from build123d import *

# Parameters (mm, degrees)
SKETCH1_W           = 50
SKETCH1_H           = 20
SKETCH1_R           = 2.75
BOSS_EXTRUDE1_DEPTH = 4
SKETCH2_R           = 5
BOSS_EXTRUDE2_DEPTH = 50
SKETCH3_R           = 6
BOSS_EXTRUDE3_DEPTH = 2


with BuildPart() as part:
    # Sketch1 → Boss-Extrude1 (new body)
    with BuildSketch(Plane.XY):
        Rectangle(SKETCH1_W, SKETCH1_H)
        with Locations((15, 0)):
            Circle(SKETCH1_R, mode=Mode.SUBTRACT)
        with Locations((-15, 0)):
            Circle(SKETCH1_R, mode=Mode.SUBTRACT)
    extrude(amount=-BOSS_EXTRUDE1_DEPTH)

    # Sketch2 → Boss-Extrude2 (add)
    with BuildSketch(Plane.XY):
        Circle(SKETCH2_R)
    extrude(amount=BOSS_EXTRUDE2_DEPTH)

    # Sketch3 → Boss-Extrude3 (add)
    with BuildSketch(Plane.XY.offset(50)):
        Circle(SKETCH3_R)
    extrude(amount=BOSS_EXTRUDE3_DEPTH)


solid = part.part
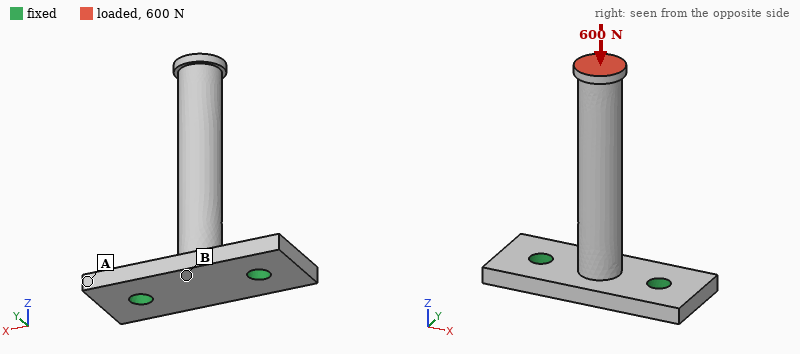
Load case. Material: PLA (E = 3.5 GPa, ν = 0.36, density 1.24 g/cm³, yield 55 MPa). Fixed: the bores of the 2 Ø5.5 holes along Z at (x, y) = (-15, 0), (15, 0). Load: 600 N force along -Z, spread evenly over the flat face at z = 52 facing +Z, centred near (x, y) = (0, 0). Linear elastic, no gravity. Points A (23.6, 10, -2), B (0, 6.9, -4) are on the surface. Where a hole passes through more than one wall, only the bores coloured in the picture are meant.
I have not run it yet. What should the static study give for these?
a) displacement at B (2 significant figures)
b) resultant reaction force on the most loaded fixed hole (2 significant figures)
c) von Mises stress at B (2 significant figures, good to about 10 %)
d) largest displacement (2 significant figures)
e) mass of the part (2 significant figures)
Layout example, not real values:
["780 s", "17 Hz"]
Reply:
["0.16 mm", "310 N", "17 MPa", "0.27 mm", "9.9 g"]
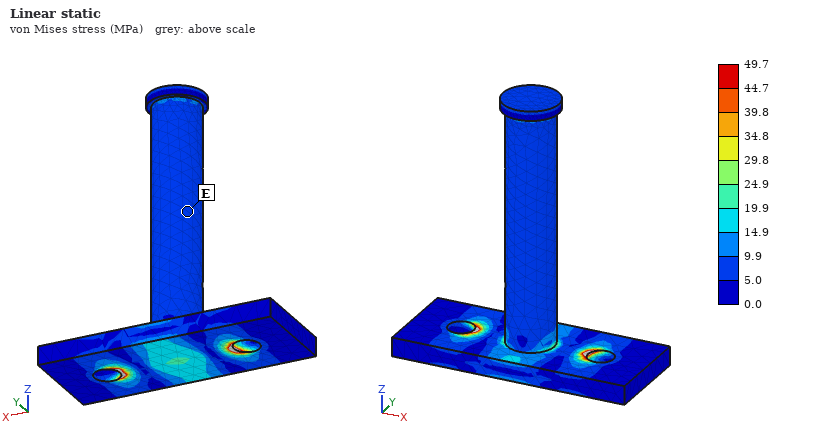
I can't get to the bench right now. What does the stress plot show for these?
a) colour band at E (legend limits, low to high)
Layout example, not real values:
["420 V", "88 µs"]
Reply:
["5.0 to 9.9 MPa"]
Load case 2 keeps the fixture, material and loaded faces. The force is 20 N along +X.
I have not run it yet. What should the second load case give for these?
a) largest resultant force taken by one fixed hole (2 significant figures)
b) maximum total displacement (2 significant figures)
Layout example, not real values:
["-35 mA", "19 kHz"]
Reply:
["55 N", "0.75 mm"]
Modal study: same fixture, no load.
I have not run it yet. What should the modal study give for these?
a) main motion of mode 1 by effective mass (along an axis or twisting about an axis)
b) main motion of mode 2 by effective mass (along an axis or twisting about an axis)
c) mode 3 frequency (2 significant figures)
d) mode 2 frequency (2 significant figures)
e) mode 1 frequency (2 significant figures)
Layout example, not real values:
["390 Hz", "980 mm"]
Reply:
["along Y", "along X", "3600 Hz", "680 Hz", "540 Hz"]
